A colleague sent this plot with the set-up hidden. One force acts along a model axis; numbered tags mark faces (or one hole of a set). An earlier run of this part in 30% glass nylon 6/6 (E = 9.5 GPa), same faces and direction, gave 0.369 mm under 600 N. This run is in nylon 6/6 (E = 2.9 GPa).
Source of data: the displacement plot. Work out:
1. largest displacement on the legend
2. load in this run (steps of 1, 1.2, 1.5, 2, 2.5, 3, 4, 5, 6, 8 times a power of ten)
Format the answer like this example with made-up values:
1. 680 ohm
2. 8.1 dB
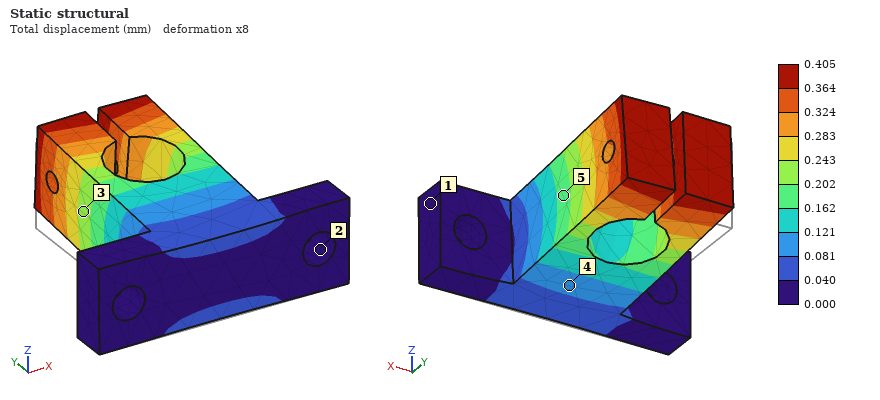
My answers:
1. 0.405 mm
2. 200 N
